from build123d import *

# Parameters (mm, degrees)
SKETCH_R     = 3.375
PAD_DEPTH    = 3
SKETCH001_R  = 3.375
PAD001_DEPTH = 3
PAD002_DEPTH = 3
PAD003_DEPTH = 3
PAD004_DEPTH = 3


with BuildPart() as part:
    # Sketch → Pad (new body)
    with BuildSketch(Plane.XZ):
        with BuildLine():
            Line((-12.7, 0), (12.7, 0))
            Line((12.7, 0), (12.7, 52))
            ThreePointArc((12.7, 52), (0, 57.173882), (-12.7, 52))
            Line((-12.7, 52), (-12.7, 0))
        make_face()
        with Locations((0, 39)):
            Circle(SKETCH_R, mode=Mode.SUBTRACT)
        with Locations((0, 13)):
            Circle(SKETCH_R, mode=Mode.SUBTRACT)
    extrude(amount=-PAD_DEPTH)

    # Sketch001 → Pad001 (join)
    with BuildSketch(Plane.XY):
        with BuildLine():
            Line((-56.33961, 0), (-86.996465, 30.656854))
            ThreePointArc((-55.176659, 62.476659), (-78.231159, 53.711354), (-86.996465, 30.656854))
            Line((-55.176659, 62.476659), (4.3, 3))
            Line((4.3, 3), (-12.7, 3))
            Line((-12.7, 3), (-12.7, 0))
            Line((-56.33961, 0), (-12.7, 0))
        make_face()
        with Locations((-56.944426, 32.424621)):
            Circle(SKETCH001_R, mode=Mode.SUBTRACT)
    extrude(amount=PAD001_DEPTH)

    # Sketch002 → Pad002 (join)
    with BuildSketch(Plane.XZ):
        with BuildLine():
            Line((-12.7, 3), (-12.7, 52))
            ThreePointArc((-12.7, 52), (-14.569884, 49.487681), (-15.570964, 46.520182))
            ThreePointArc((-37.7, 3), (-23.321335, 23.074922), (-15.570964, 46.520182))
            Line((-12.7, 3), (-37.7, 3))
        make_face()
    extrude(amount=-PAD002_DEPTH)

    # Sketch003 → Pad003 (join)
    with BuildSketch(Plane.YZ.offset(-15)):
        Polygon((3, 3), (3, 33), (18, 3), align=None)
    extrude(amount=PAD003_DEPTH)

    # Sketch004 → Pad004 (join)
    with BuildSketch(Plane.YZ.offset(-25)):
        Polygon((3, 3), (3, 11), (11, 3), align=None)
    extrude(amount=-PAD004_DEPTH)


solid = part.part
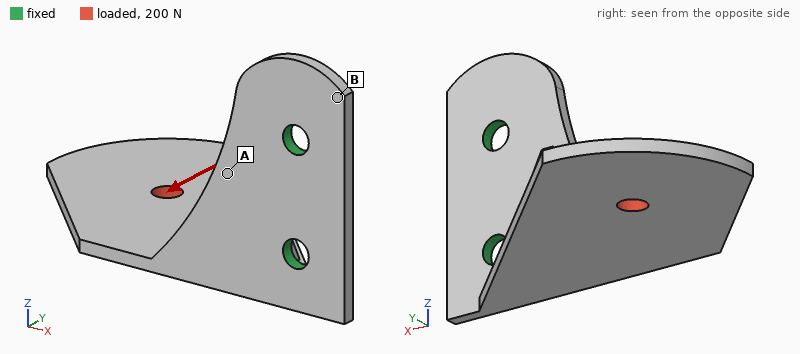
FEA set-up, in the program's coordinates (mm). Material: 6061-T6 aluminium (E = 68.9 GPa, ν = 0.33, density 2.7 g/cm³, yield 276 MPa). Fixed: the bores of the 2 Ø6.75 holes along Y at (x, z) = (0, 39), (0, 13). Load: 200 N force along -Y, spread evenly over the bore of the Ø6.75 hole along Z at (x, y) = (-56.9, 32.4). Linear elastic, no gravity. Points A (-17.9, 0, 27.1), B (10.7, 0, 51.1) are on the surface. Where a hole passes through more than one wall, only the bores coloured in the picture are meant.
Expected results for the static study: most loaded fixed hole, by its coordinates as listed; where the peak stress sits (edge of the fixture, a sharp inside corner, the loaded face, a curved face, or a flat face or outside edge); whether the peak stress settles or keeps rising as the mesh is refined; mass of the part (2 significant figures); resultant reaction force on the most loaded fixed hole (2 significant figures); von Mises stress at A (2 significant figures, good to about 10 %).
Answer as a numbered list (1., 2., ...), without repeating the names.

1. (0, 13)
2. edge of the fixture
3. keeps rising
4. 43 g
5. 340 N
6. 60 MPa
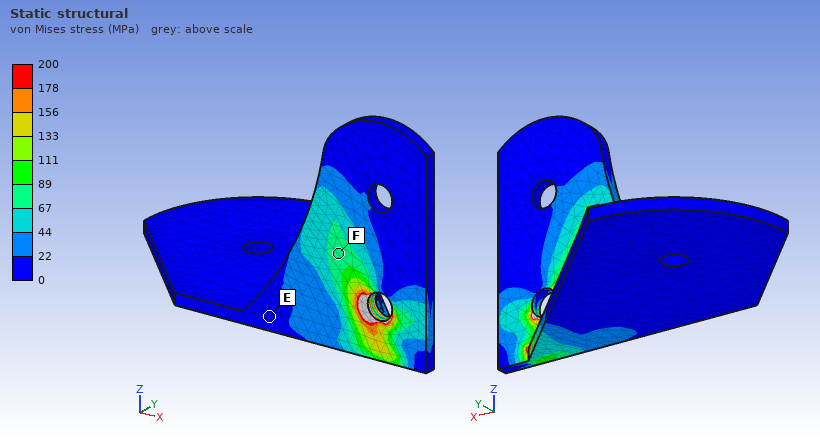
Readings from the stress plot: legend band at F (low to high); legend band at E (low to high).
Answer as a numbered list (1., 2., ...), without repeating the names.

1. 67 to 89 MPa
2. 0 to 22 MPa
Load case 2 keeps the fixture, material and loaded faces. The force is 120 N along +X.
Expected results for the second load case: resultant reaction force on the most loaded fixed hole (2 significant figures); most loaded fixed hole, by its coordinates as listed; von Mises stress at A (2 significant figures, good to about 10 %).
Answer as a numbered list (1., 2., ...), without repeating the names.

1. 150 N
2. (0, 13)
3. 20 MPa
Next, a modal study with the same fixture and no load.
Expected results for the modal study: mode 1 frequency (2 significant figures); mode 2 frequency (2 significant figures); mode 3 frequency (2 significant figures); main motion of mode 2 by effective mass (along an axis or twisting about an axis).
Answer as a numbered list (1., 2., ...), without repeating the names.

1. 400 Hz
2. 510 Hz
3. 1600 Hz
4. along Y
